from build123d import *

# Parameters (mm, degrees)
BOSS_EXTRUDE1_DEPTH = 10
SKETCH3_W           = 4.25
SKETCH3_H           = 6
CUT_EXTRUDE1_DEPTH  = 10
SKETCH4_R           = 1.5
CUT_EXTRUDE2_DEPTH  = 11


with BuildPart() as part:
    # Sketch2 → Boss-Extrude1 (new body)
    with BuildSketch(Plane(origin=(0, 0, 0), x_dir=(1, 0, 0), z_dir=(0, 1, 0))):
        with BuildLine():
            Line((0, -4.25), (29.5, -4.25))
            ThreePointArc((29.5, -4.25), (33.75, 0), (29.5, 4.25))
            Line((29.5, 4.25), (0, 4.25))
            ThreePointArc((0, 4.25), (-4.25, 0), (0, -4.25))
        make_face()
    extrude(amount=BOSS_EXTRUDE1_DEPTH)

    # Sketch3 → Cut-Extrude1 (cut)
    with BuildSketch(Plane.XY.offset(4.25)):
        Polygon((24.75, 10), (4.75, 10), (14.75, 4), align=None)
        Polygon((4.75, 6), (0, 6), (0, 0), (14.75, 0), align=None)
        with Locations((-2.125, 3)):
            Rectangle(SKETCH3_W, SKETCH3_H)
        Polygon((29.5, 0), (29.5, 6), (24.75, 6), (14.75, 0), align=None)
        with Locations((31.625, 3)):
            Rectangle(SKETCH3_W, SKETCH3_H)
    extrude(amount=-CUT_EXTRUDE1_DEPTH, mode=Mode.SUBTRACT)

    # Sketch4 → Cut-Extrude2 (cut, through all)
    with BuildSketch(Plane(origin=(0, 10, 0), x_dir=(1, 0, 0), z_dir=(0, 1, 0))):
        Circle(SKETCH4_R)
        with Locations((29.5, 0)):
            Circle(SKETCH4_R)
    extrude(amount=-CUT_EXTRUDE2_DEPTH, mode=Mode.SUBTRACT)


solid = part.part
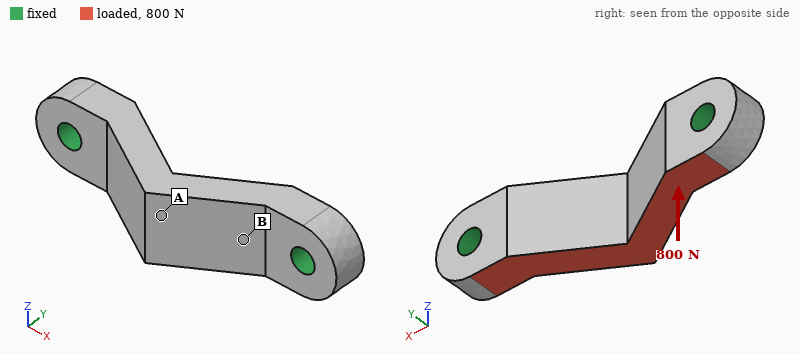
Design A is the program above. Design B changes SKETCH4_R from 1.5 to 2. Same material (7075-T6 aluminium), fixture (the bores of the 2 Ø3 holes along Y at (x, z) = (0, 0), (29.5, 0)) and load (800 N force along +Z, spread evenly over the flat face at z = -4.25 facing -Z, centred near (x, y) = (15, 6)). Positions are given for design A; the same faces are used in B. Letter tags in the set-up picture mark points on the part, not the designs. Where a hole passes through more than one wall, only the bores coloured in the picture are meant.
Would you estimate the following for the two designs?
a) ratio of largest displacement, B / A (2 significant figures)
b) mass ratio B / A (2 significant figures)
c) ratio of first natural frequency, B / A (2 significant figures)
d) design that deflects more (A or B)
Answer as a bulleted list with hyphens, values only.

- 0.81
- 0.96
- 1.1
- A
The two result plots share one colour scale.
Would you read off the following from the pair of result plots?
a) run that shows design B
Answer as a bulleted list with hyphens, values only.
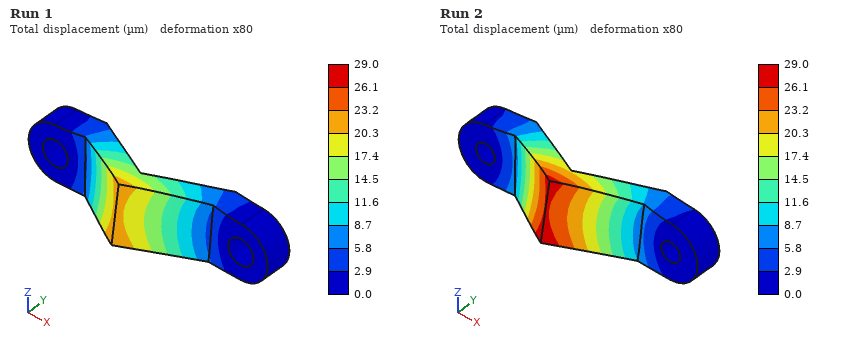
- Run 1
